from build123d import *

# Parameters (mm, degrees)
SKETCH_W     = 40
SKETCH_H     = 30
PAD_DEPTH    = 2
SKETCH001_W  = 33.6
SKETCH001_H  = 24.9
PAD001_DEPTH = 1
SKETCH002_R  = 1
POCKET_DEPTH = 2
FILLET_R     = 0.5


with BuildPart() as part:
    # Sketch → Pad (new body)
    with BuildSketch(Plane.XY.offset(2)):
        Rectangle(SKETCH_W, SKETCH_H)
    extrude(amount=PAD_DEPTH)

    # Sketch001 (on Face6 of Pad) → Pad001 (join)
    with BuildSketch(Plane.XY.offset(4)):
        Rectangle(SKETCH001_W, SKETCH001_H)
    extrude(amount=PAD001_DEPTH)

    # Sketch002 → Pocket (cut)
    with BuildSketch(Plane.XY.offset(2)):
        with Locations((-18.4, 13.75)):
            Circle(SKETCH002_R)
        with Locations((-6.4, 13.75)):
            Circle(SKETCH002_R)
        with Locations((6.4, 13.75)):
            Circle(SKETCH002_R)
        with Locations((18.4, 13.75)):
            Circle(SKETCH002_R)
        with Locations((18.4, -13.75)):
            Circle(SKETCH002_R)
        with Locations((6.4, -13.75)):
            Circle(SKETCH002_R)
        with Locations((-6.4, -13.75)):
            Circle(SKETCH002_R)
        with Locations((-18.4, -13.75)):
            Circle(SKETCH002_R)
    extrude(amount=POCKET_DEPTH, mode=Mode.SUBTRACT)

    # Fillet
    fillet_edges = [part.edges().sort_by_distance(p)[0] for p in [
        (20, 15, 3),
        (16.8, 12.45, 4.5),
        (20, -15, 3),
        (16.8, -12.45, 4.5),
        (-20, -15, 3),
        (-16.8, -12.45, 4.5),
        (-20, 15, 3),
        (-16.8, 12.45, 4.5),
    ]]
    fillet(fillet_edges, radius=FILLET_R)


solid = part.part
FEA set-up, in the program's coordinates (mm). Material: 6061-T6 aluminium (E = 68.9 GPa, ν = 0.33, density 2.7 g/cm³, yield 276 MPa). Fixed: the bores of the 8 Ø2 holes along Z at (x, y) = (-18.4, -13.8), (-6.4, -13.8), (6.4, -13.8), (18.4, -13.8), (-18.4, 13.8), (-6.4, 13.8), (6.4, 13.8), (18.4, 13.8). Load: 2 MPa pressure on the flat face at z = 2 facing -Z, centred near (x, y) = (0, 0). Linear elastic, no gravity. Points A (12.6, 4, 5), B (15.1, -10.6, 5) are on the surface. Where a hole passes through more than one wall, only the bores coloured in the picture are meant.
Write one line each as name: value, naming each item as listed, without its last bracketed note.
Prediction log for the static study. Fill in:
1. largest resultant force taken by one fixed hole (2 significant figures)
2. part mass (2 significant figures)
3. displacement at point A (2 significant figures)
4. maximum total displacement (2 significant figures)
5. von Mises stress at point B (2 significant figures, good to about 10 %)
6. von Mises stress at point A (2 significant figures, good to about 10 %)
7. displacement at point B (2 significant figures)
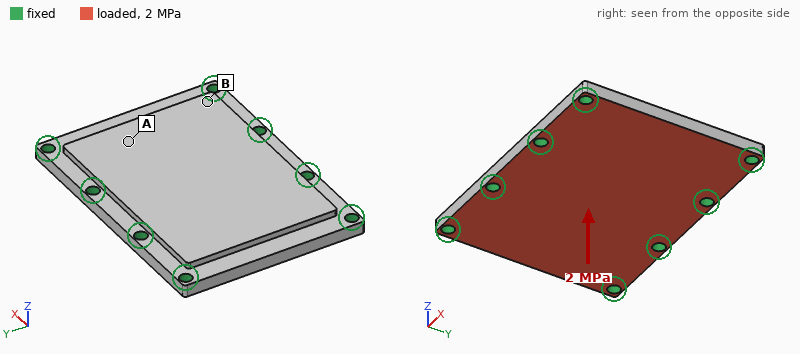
largest resultant force taken by one fixed hole: 430 N
part mass: 8.6 g
displacement at point A: 36 µm
maximum total displacement: 50 µm
von Mises stress at point B: 27 MPa
von Mises stress at point A: 58 MPa
displacement at point B: 14 µm
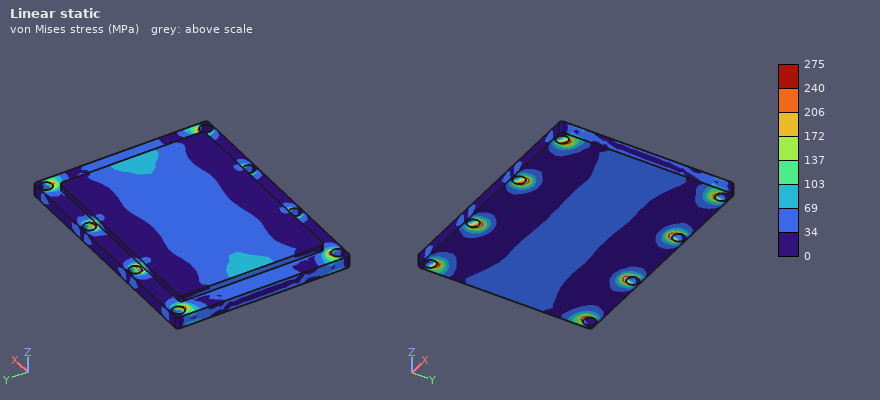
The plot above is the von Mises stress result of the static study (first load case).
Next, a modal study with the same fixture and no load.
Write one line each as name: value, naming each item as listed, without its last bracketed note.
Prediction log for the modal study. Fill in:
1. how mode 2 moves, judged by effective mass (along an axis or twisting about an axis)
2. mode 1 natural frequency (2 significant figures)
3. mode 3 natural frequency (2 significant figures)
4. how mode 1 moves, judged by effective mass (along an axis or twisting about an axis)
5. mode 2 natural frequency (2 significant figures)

how mode 2 moves, judged by effective mass: twisting about Y
mode 1 natural frequency: 14 kHz
mode 3 natural frequency: 24 kHz
how mode 1 moves, judged by effective mass: along Z
mode 2 natural frequency: 17 kHz
